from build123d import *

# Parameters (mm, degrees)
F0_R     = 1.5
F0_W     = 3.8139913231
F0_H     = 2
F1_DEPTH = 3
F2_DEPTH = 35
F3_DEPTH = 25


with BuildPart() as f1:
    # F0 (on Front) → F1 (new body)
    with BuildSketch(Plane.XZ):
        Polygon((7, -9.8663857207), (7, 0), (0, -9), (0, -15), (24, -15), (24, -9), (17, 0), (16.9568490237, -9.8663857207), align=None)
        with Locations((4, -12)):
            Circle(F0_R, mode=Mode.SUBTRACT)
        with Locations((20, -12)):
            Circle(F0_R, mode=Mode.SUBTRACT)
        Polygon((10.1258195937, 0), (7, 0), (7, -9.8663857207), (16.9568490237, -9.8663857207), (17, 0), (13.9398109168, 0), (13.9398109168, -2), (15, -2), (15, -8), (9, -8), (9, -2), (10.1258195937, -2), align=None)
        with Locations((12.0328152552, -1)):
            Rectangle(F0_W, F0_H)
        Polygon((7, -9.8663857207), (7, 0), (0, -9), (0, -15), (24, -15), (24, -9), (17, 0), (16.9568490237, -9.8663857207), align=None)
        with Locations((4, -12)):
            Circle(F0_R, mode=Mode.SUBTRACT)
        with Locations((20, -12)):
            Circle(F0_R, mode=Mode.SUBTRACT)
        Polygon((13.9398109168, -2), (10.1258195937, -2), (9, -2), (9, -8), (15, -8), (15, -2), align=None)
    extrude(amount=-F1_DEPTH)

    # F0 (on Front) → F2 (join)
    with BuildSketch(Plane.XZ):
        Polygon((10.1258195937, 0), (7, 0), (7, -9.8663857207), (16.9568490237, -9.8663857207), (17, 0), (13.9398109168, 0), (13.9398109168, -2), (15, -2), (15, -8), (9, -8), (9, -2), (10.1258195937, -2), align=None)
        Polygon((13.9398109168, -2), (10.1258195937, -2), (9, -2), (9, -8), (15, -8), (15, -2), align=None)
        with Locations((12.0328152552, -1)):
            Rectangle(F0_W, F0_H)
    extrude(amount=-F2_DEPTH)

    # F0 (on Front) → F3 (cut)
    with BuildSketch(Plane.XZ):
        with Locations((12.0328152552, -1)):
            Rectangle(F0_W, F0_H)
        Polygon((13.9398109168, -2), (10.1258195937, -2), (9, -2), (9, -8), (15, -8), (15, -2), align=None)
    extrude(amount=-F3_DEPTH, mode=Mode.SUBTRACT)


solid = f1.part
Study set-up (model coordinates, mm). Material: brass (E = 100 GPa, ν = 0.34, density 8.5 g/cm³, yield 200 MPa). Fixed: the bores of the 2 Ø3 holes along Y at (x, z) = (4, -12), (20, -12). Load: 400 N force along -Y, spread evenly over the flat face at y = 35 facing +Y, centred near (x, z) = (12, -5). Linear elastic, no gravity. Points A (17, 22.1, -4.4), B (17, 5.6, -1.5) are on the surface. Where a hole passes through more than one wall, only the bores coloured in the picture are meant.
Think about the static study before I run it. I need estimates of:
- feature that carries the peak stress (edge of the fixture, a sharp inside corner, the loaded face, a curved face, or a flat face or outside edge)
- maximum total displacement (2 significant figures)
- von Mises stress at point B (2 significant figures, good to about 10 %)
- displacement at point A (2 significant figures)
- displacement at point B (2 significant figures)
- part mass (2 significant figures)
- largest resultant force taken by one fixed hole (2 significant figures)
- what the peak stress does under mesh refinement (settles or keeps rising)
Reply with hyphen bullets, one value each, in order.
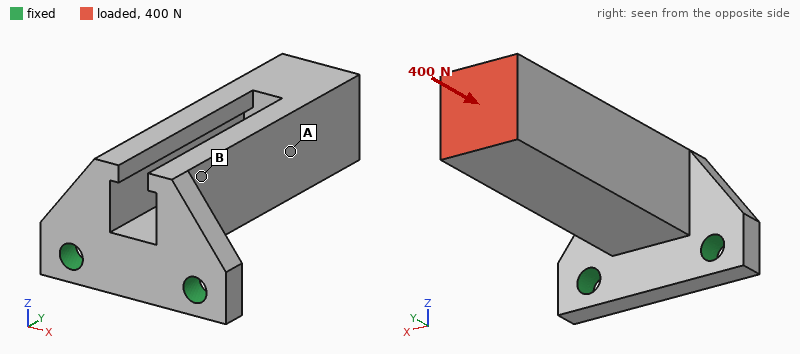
- edge of the fixture
- 84 µm
- 22 MPa
- 51 µm
- 24 µm
- 25 g
- 200 N
- keeps rising
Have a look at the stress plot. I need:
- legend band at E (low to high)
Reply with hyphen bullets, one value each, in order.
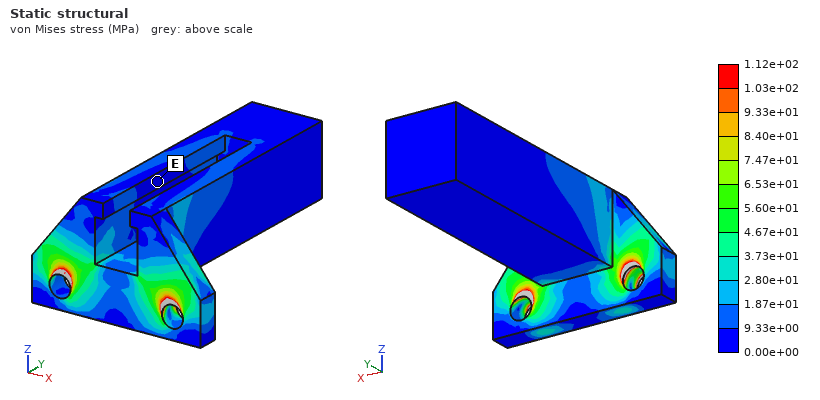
- 0.00e+00 to 9.33e+00 MPa
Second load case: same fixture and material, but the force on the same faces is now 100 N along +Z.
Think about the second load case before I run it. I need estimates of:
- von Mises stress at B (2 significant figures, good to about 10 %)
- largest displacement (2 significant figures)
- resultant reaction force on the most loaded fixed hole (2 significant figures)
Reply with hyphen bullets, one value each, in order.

- 38 MPa
- 0.16 mm
- 55 N
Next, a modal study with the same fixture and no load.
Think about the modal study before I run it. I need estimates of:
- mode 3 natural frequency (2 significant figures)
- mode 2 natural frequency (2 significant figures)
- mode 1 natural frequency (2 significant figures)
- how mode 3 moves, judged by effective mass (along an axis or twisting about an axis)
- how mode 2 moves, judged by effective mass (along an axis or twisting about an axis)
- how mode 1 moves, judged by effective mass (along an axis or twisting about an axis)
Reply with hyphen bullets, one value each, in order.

- 5400 Hz
- 2500 Hz
- 1400 Hz
- twisting about Y
- along X
- along Z
